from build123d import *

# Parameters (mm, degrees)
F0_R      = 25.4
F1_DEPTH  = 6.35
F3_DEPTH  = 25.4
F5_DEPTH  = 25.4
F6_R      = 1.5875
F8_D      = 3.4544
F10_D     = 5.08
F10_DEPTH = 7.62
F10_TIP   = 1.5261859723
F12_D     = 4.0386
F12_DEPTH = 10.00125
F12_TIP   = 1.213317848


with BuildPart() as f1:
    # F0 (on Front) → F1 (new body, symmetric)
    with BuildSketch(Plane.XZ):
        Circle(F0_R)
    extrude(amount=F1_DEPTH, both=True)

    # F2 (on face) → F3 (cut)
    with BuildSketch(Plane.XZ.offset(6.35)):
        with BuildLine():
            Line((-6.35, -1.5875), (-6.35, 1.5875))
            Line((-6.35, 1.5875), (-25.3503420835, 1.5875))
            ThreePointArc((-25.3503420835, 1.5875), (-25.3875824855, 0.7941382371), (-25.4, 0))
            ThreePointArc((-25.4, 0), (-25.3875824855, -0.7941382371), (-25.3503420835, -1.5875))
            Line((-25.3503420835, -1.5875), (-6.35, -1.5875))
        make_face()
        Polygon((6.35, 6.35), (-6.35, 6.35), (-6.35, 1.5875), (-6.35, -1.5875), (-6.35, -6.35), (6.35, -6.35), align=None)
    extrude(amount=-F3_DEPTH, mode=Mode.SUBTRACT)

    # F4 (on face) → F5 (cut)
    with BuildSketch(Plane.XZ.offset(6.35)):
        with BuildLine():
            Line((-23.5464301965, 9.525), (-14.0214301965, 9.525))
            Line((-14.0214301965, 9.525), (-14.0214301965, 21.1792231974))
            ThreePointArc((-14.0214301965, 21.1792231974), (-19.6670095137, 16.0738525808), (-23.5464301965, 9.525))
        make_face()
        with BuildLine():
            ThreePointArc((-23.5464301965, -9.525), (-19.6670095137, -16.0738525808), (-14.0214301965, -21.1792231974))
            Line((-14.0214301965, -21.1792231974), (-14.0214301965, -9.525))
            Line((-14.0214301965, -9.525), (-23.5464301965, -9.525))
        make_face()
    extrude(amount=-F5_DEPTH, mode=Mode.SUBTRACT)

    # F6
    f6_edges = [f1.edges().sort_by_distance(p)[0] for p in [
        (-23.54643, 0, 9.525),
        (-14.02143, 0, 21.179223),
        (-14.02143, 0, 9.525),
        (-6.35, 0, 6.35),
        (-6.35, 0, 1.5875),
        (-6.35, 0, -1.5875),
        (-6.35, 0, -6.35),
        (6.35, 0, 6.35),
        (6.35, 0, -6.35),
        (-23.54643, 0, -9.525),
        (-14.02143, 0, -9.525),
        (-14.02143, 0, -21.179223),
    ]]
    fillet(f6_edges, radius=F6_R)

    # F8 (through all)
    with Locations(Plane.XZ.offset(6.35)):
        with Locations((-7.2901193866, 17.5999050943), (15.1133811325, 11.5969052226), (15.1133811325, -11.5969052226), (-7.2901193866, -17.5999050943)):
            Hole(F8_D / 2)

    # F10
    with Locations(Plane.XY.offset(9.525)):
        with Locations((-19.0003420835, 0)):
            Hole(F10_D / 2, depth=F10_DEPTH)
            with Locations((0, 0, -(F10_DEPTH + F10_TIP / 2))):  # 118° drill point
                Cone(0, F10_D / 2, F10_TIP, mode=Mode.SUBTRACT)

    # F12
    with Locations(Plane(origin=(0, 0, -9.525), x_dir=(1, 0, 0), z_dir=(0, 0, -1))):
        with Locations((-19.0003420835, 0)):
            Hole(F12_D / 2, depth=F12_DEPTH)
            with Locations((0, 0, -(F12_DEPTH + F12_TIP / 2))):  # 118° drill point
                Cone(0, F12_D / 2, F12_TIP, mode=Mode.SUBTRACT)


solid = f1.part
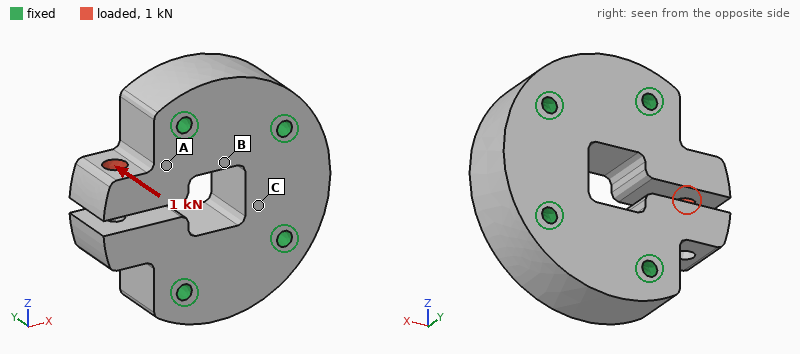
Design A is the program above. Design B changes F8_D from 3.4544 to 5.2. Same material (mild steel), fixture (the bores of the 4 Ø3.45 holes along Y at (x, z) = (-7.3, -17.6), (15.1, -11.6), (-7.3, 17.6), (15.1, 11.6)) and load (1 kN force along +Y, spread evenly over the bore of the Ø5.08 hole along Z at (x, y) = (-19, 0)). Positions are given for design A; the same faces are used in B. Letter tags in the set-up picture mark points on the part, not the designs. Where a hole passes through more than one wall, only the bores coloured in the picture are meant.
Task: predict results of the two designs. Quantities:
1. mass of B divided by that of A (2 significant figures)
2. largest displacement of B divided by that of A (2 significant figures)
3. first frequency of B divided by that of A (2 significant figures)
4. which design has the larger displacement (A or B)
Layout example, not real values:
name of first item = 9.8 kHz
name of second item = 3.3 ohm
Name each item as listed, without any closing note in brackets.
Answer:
mass of B divided by that of A = 0.97
largest displacement of B divided by that of A = 0.90
first frequency of B divided by that of A = 1.1
which design has the larger displacement = A
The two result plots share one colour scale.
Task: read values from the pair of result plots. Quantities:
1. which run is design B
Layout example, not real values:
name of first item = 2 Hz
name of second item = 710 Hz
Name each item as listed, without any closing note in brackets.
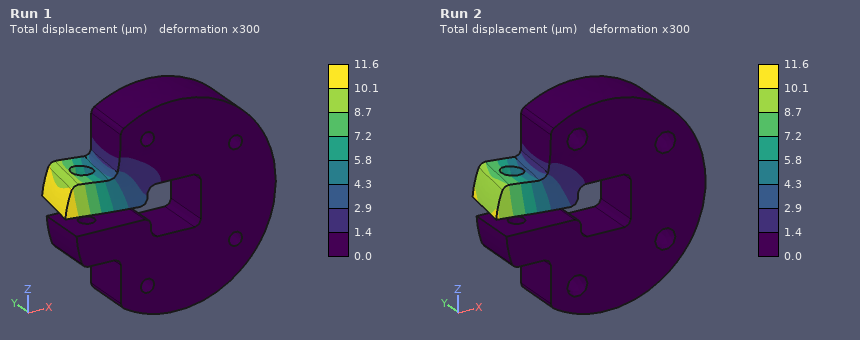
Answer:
which run is design B = Run 2
